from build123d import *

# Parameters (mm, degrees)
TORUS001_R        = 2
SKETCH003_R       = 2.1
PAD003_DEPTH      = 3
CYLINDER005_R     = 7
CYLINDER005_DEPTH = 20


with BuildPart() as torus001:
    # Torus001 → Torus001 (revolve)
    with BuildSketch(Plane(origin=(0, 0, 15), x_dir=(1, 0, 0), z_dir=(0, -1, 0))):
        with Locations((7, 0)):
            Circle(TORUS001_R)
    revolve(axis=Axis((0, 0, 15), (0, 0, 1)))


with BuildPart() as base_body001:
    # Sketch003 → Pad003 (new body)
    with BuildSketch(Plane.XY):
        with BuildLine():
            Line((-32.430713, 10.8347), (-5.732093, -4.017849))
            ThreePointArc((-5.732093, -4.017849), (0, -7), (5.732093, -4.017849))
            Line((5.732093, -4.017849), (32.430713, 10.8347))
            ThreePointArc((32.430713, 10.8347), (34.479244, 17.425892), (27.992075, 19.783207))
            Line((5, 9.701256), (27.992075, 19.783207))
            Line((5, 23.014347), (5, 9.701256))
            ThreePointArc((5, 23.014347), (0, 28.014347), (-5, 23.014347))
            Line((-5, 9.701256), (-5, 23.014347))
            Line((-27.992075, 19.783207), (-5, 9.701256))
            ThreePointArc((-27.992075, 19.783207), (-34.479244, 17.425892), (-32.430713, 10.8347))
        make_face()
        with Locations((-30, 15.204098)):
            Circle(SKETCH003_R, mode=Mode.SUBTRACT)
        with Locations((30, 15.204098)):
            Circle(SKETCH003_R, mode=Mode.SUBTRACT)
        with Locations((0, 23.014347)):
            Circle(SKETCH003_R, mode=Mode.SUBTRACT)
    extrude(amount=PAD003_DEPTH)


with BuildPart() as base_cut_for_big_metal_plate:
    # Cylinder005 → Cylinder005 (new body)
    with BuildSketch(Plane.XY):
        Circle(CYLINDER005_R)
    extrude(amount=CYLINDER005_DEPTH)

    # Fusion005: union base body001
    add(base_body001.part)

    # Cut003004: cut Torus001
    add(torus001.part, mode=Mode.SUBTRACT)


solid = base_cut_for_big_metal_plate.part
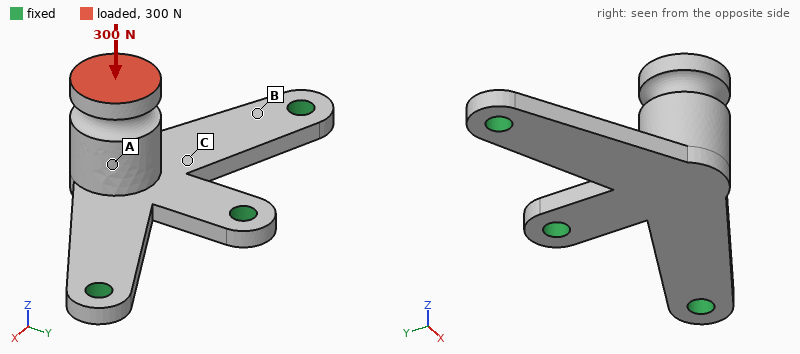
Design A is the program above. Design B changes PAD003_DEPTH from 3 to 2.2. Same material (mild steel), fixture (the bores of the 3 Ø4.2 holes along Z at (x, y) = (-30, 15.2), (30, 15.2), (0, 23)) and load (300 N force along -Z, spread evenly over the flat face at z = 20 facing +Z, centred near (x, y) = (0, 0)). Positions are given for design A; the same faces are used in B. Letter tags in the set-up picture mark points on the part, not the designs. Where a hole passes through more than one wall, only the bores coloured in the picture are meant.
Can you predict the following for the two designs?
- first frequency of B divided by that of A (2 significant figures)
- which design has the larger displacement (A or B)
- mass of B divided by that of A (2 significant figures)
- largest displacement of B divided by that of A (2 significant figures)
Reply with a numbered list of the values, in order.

1. 0.65
2. B
3. 0.87
4. 2.4
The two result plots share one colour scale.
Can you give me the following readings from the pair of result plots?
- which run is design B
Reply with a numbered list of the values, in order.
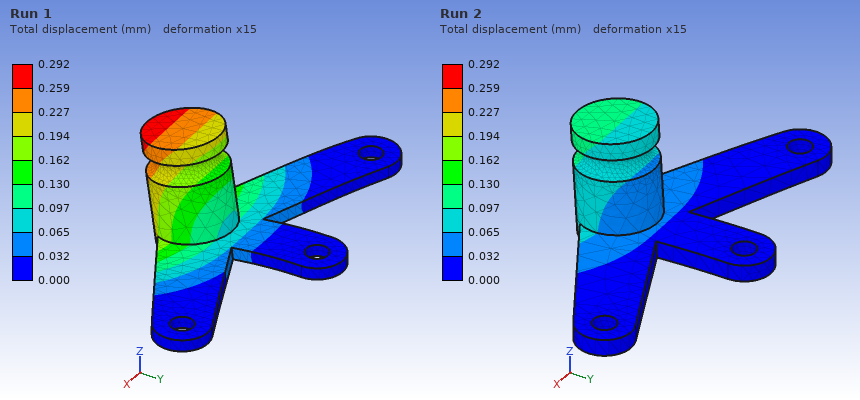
1. Run 1
